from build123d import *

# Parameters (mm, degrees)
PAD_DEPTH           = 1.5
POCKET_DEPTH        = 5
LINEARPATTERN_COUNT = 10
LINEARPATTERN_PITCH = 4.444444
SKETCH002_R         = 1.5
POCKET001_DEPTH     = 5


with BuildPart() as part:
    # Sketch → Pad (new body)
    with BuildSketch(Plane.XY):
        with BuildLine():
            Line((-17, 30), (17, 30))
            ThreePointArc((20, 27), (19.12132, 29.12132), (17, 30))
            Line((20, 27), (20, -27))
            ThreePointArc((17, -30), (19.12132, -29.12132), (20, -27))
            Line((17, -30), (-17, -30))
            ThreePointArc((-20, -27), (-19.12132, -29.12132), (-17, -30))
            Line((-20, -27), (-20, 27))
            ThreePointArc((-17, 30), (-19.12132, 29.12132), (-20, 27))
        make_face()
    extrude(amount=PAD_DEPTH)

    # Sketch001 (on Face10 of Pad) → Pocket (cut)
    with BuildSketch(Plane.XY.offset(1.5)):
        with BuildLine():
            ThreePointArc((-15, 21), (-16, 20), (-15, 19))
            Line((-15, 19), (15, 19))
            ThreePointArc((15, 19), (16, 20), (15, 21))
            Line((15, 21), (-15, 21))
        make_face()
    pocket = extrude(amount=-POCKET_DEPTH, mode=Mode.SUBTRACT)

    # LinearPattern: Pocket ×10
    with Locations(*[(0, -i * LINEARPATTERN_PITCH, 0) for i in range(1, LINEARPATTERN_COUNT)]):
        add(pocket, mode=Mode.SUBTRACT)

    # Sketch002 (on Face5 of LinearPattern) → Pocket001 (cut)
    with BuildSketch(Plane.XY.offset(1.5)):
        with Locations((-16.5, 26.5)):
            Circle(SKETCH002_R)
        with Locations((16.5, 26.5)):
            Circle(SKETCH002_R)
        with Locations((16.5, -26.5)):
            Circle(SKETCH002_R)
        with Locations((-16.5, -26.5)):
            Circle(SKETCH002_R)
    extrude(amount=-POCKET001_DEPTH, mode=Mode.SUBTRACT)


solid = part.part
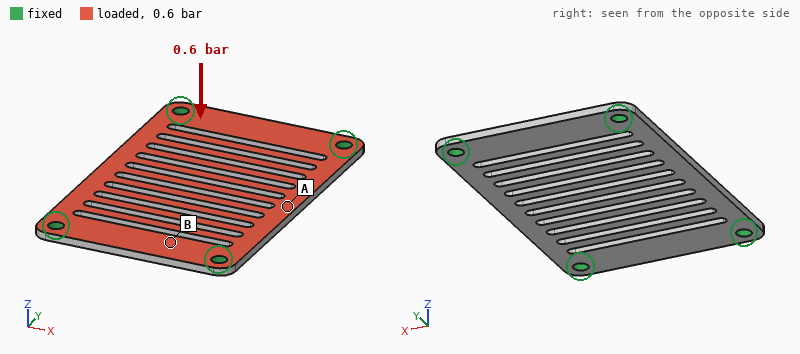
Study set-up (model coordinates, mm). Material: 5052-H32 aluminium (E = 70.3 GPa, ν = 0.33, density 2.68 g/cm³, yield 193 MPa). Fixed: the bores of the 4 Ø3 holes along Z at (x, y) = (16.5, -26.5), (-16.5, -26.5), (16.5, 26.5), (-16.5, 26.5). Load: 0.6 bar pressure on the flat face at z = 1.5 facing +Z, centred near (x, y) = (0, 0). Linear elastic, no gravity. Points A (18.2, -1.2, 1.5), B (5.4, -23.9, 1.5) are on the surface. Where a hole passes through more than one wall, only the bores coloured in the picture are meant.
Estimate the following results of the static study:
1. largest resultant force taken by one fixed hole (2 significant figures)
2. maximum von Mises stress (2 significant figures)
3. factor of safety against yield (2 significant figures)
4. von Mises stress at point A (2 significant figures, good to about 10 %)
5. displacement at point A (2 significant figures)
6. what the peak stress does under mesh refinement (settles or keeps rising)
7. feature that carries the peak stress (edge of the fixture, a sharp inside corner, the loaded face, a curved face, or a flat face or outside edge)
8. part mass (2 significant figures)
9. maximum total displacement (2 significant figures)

26 N
98 MPa
2.0
45 MPa
0.13 mm
settles
the loaded face
7.0 g
0.18 mm
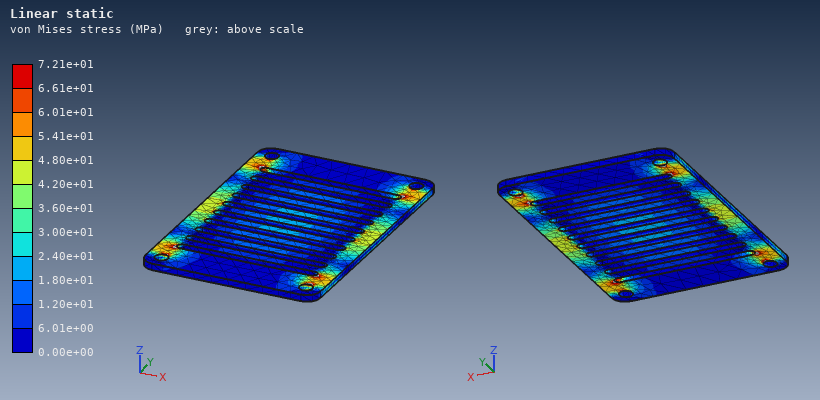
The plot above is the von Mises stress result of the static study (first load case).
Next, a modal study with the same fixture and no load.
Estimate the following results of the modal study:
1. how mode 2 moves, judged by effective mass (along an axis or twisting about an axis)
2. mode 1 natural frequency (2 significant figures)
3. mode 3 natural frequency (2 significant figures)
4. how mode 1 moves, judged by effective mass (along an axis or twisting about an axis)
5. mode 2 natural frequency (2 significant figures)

twisting about Y
1800 Hz
3600 Hz
along Z
3200 Hz
